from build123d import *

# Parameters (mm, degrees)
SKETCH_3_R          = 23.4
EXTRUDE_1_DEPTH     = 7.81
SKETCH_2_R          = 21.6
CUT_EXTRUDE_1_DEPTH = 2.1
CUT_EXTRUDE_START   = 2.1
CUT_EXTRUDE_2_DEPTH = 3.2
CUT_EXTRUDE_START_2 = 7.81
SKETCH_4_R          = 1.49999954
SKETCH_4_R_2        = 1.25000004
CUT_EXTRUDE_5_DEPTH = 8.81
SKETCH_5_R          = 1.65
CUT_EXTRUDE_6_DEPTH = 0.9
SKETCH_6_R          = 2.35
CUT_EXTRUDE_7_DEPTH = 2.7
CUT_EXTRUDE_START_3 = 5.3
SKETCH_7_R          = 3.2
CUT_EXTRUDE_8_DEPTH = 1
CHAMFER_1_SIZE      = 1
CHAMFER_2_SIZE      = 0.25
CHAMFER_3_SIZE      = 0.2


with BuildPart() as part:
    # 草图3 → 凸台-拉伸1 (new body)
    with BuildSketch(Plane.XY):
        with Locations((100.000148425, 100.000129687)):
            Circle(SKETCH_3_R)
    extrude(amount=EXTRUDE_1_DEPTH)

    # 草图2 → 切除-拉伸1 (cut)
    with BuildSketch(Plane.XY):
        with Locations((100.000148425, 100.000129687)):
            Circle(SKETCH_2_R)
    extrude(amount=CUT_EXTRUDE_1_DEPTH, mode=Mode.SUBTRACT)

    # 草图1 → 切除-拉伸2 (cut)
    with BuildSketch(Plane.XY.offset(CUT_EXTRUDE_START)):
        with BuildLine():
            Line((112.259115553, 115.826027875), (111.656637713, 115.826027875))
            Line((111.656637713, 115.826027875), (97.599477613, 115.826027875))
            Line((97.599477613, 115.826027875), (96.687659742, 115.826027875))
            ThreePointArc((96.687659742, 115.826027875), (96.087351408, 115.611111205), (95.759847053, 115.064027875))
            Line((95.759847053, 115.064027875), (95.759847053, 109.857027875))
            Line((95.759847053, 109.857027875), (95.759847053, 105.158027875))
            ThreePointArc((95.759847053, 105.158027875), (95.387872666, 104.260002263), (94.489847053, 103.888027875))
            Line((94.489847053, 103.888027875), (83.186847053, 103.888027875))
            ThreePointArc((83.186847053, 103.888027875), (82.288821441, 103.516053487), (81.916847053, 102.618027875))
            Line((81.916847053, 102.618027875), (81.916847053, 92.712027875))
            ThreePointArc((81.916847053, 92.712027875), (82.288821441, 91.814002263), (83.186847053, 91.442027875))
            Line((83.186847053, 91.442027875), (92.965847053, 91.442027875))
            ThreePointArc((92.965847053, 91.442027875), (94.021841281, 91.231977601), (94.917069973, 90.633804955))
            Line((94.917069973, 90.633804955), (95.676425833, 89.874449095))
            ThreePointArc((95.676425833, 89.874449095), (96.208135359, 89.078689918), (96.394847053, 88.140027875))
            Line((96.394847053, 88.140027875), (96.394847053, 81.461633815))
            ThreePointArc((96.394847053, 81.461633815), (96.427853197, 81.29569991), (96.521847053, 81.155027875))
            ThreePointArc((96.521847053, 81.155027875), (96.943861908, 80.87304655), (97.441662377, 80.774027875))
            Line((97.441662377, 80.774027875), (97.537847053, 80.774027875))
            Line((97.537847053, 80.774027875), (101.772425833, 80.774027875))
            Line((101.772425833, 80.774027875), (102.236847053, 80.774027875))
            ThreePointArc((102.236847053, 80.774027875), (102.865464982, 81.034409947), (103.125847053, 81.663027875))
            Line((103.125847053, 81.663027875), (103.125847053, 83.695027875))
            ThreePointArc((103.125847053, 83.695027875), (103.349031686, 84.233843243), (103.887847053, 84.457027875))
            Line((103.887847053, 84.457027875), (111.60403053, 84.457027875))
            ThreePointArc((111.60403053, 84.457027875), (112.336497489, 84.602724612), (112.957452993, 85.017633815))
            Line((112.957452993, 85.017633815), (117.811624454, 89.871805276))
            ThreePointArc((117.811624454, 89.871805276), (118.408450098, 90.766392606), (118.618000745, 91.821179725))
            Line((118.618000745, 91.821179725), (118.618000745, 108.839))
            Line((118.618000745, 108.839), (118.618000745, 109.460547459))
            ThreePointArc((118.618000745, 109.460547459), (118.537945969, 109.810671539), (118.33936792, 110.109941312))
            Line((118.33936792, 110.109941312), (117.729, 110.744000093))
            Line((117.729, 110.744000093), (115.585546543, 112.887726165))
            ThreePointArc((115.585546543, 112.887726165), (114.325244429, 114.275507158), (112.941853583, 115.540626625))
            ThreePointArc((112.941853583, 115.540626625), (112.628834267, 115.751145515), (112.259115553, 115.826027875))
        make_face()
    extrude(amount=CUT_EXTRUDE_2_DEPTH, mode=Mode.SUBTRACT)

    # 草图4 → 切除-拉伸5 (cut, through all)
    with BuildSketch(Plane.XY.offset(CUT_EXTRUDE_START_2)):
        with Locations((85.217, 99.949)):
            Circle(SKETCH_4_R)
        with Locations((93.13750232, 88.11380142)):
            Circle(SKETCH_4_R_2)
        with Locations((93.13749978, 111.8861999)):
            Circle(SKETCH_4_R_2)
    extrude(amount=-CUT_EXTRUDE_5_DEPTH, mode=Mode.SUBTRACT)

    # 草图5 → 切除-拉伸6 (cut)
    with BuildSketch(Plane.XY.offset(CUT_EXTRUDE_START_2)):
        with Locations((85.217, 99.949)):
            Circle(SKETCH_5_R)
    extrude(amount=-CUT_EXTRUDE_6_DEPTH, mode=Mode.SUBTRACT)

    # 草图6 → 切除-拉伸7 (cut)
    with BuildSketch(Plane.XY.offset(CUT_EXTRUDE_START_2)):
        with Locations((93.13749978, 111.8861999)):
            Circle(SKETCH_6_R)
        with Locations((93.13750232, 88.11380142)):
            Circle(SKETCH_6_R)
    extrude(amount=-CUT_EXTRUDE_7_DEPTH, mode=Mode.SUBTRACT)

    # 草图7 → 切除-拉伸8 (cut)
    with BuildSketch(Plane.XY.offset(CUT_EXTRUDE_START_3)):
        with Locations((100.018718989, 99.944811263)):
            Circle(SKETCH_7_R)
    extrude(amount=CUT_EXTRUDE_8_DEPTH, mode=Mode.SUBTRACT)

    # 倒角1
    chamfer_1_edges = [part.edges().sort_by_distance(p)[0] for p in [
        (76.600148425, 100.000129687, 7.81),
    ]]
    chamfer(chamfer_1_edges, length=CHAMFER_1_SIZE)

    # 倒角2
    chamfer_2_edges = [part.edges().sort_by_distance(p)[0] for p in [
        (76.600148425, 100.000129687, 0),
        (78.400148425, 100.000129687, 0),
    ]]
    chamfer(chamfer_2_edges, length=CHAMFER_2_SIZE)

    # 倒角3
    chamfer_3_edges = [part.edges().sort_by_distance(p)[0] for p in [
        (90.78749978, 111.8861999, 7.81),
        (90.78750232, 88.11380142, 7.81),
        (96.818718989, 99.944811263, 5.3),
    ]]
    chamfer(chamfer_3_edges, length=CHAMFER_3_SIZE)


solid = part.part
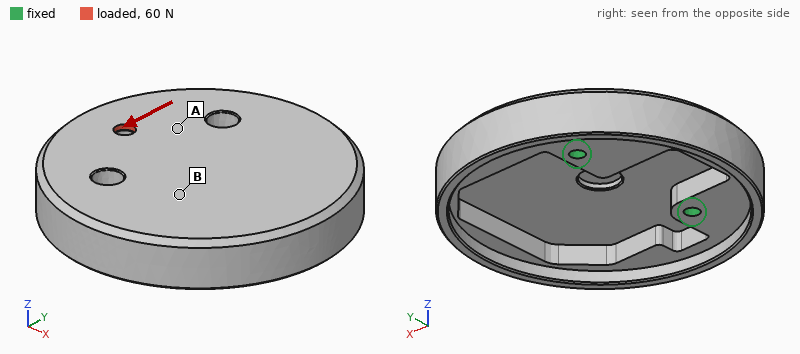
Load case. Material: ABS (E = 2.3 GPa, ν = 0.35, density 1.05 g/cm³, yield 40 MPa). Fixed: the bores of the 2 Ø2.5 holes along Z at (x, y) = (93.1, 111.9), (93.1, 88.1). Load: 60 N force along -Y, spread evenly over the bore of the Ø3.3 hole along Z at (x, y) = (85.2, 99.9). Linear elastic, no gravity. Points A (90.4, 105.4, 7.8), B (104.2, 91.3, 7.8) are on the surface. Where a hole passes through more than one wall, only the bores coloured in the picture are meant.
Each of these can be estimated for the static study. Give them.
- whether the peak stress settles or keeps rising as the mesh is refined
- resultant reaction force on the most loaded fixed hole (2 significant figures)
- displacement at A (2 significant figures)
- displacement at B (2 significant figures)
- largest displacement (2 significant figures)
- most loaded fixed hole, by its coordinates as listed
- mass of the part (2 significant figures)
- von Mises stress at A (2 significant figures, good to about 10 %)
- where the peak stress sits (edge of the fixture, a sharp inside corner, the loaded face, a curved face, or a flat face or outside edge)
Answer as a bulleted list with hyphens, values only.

- keeps rising
- 39 N
- 6.5 µm
- 2.6 µm
- 17 µm
- (93.1, 111.9)
- 7.7 g
- 0.95 MPa
- a sharp inside corner
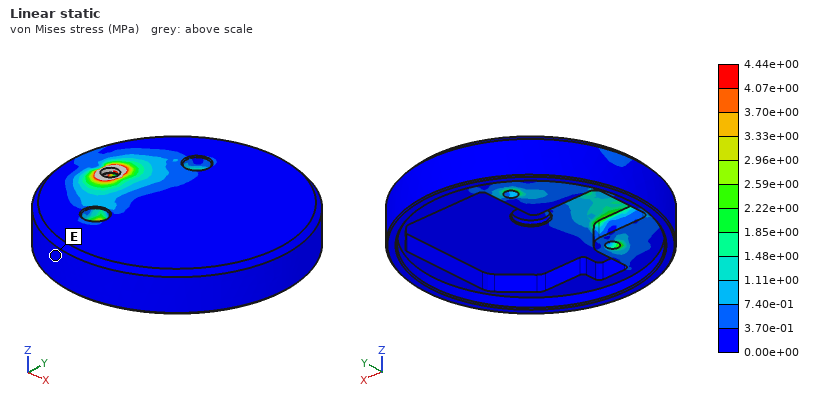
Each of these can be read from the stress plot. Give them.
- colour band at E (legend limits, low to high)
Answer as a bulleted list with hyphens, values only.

- 0.00e+00 to 3.70e-01 MPa
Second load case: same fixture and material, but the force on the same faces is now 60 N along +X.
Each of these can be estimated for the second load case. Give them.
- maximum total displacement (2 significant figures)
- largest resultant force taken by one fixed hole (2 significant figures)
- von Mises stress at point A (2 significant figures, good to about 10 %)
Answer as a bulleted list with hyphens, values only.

- 94 µm
- 31 N
- 1.3 MPa
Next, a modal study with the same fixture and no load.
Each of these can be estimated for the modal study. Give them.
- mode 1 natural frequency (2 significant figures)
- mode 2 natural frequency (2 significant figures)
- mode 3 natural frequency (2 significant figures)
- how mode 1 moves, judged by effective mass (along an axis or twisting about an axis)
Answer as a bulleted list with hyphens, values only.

- 840 Hz
- 2000 Hz
- 3000 Hz
- along Z
